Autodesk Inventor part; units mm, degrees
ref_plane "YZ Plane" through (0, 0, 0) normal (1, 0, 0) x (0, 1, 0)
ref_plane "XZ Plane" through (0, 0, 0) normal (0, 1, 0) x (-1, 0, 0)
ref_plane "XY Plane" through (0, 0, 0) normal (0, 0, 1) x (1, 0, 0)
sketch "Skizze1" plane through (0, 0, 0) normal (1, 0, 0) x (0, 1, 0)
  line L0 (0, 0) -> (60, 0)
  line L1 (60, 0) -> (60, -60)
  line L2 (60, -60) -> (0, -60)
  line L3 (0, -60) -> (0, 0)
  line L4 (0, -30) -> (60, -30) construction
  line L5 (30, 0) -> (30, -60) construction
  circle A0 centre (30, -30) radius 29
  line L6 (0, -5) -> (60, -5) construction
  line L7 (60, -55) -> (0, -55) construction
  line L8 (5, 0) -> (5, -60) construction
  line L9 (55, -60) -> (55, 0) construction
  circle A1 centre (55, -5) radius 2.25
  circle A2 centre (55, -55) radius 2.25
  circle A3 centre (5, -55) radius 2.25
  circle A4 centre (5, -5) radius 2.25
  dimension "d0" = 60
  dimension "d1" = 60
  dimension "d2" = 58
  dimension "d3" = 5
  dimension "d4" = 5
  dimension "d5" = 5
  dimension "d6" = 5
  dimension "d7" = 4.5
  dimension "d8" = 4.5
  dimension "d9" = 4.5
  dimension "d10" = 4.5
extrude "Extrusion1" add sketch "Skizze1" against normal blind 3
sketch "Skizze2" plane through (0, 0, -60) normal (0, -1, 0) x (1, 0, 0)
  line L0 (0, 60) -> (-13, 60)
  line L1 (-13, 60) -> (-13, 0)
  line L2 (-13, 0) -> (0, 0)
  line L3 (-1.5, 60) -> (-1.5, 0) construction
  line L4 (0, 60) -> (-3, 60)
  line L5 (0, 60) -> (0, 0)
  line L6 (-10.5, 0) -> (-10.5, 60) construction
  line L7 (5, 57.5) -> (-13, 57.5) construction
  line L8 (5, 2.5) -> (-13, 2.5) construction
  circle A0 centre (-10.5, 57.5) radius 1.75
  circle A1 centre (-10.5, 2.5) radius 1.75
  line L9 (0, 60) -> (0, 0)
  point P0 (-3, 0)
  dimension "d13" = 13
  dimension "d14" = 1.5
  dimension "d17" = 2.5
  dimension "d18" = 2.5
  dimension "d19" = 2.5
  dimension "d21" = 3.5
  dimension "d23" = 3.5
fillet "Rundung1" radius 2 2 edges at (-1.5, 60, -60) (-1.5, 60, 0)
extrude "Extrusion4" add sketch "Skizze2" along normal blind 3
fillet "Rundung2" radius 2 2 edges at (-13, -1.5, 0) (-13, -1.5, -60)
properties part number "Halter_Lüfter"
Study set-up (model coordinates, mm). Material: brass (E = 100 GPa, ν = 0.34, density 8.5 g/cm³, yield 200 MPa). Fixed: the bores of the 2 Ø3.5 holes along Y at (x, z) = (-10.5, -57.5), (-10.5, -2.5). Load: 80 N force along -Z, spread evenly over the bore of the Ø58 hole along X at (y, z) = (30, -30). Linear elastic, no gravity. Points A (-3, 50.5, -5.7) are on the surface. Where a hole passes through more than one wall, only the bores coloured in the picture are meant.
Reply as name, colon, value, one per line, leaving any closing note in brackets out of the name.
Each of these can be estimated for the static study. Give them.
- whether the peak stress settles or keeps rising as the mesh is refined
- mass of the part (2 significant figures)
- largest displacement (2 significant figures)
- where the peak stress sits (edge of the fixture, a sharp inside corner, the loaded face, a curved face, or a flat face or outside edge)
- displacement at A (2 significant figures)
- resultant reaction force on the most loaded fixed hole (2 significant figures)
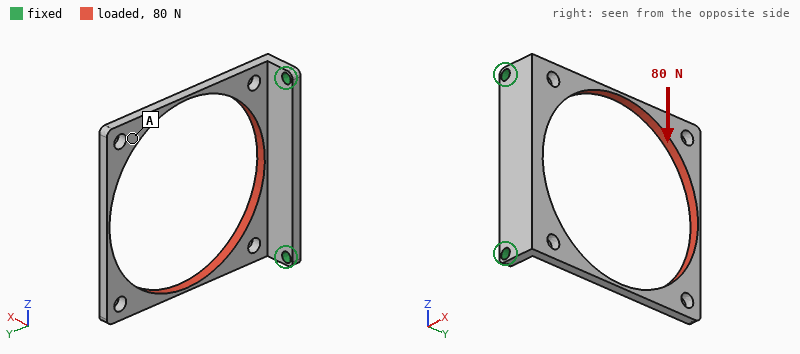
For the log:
whether the peak stress settles or keeps rising as the mesh is refined: keeps rising
mass of the part: 42 g
largest displacement: 0.19 mm
where the peak stress sits: a sharp inside corner
displacement at A: 0.18 mm
resultant reaction force on the most loaded fixed hole: 60 N
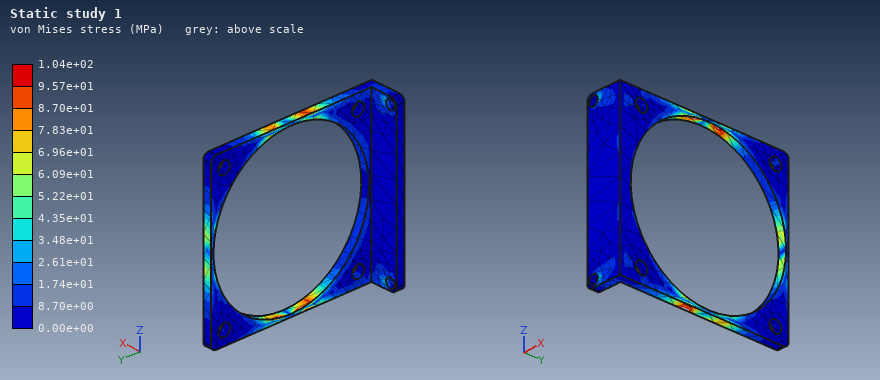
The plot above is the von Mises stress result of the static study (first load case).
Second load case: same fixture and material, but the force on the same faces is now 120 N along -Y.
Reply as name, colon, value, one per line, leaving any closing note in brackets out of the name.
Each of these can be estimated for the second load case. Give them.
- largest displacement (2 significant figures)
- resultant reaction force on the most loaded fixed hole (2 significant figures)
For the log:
largest displacement: 90 µm
resultant reaction force on the most loaded fixed hole: 60 N
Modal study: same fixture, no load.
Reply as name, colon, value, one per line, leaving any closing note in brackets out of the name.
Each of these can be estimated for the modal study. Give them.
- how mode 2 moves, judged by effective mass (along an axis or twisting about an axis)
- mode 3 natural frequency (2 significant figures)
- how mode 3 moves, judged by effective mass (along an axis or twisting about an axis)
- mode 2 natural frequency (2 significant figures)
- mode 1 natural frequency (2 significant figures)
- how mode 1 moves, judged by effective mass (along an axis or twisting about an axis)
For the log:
how mode 2 moves, judged by effective mass: twisting about Y
mode 3 natural frequency: 700 Hz
how mode 3 moves, judged by effective mass: along Z
mode 2 natural frequency: 470 Hz
mode 1 natural frequency: 250 Hz
how mode 1 moves, judged by effective mass: along X
